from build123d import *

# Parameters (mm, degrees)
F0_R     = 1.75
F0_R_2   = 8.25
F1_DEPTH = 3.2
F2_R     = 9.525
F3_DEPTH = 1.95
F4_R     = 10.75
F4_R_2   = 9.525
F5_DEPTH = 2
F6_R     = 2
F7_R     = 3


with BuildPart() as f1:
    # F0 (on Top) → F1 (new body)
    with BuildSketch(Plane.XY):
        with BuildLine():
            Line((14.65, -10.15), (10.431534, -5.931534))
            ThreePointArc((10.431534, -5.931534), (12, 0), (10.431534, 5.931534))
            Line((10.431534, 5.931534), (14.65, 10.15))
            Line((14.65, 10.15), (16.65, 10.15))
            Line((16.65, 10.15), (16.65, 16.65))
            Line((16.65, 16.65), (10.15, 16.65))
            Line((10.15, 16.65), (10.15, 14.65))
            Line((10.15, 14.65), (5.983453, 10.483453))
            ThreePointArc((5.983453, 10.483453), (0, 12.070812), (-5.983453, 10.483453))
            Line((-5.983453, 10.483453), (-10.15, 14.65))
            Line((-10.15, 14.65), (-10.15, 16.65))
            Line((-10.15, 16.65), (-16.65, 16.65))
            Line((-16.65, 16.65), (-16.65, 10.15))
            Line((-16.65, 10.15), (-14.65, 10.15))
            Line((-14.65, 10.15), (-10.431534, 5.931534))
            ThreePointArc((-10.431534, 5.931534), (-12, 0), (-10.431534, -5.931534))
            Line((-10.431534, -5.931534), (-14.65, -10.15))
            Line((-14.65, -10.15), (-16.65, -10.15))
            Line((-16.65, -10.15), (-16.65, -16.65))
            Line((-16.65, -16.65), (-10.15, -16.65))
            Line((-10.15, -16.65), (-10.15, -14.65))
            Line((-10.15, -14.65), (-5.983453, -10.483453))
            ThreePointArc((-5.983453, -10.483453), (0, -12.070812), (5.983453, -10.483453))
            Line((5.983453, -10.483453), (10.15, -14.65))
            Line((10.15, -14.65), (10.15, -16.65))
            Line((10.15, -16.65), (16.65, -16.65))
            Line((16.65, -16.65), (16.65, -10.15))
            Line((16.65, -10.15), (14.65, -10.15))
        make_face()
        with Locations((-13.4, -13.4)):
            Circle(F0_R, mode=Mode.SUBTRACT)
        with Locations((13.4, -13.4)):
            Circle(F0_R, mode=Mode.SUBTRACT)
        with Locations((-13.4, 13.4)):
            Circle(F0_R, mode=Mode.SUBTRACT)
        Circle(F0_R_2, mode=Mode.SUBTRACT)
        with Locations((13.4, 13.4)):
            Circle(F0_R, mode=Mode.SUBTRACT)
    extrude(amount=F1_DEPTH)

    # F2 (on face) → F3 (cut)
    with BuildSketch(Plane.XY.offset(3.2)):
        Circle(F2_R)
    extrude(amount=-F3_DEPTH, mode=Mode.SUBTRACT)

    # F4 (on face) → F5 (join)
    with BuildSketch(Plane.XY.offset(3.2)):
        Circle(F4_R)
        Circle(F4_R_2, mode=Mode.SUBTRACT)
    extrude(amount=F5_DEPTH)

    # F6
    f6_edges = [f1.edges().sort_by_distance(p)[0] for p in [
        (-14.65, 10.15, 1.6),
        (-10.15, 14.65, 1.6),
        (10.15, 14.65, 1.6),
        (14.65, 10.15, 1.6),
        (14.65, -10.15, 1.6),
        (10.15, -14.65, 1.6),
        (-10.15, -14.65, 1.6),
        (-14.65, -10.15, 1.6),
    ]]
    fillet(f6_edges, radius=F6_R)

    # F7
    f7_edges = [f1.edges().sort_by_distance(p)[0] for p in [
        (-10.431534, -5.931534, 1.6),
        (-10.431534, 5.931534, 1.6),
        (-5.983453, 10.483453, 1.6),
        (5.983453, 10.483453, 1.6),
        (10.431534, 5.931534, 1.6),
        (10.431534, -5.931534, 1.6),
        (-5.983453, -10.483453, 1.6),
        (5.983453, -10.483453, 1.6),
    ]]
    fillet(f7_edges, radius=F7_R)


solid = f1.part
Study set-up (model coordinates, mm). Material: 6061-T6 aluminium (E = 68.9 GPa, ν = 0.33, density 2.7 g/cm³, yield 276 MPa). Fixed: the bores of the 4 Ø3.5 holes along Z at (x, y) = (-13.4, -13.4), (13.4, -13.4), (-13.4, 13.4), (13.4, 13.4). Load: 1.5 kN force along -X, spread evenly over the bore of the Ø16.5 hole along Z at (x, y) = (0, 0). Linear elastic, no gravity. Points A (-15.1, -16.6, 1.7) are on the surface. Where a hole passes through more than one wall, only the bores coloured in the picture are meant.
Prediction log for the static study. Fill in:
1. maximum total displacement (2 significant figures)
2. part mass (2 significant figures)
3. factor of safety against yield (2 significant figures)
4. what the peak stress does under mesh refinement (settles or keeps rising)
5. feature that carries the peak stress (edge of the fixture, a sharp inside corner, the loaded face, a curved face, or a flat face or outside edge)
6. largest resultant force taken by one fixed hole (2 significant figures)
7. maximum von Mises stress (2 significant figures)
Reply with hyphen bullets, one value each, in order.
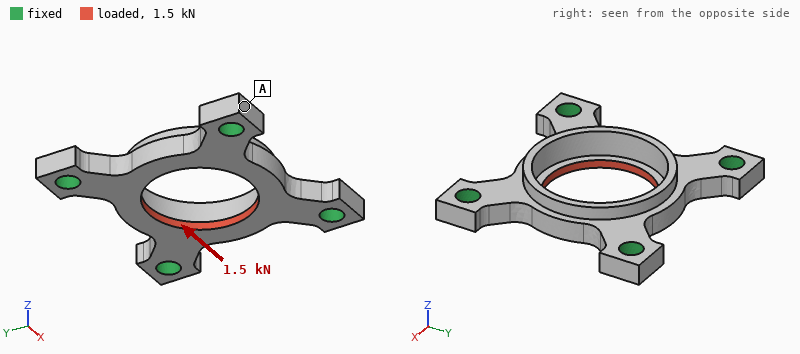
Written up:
- 19 µm
- 4.2 g
- 2.9
- settles
- the loaded face
- 420 N
- 96 MPa
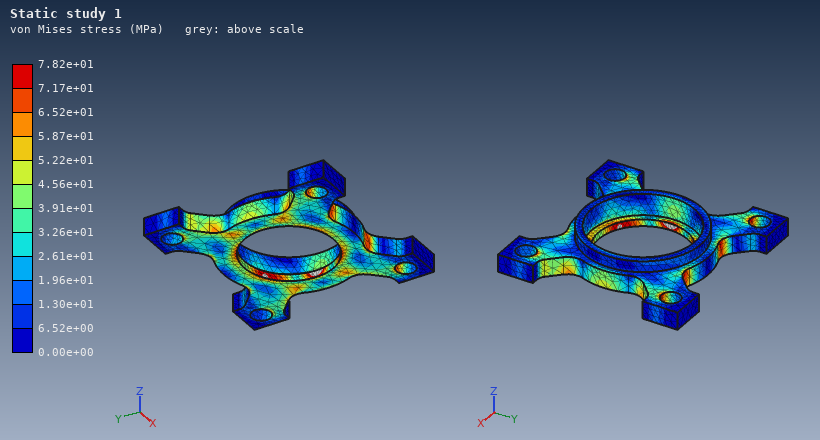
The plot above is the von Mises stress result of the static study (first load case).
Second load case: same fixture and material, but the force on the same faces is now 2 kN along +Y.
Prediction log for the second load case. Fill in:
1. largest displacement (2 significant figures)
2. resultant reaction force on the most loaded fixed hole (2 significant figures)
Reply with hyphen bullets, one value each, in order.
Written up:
- 25 µm
- 560 N
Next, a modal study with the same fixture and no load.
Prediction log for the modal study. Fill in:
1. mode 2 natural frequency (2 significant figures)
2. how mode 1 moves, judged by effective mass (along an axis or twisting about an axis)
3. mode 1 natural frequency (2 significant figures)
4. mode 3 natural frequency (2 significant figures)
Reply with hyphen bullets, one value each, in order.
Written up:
- 27 kHz
- along Z
- 22 kHz
- 27 kHz
